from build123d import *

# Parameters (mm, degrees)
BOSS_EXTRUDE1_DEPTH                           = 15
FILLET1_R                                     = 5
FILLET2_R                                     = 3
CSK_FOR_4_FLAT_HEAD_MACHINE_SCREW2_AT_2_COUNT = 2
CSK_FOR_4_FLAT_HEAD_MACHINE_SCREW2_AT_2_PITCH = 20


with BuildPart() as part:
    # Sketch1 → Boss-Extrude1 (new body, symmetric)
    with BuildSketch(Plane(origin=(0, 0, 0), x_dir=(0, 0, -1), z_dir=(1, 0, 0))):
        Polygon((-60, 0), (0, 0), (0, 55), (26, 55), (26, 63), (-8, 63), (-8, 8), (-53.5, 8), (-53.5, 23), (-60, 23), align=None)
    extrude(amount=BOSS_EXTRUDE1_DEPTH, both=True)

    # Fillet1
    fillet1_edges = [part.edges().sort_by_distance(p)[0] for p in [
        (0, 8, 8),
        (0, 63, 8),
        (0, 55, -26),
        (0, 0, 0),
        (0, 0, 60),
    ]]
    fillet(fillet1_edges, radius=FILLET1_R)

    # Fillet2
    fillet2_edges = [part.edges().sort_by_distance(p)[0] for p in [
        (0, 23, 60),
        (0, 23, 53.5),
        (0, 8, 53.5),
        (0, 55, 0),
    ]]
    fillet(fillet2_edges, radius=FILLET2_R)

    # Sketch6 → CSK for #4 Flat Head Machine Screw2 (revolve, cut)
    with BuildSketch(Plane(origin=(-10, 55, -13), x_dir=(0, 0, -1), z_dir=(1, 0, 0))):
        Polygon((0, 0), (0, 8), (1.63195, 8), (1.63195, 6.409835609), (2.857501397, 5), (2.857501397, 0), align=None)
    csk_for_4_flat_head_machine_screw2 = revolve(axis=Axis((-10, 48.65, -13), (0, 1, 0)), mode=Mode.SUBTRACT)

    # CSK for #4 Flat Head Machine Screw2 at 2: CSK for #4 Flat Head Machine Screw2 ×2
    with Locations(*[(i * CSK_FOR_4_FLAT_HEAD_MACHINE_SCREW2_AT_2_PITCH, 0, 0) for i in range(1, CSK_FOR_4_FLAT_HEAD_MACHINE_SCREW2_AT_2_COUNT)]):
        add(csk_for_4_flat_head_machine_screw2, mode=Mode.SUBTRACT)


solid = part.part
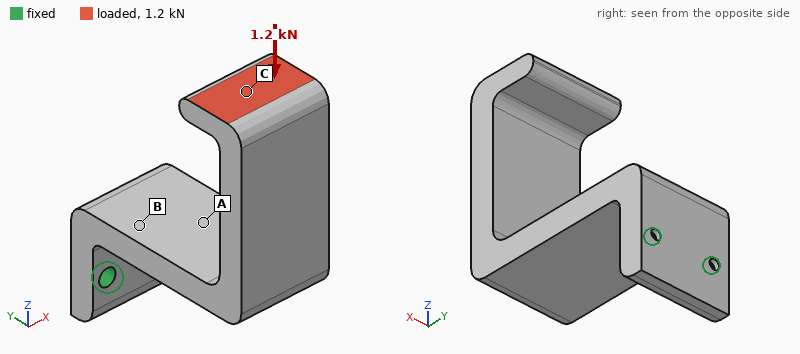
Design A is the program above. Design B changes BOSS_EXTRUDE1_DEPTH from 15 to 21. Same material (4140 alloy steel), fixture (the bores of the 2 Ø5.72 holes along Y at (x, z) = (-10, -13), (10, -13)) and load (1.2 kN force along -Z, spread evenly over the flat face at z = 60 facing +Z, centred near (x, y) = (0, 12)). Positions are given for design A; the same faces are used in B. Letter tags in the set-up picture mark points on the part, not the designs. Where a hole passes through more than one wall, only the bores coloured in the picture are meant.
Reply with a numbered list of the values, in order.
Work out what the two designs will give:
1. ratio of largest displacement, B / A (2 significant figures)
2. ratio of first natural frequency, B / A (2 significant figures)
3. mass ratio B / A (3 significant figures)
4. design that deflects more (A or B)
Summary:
1. 0.73
2. 0.99
3. 1.40
4. A
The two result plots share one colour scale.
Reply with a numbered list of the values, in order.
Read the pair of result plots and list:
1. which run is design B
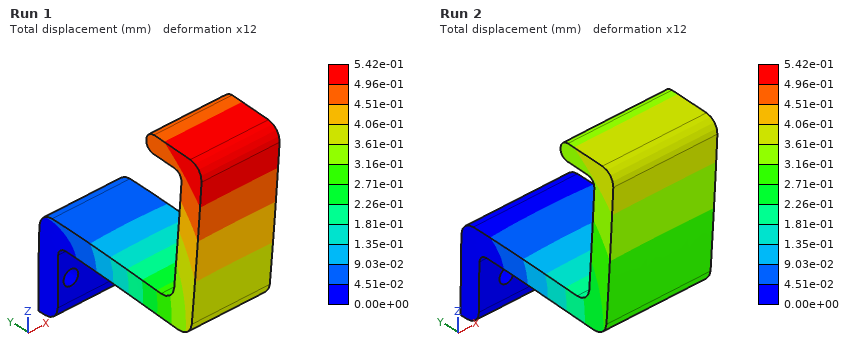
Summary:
1. Run 2
